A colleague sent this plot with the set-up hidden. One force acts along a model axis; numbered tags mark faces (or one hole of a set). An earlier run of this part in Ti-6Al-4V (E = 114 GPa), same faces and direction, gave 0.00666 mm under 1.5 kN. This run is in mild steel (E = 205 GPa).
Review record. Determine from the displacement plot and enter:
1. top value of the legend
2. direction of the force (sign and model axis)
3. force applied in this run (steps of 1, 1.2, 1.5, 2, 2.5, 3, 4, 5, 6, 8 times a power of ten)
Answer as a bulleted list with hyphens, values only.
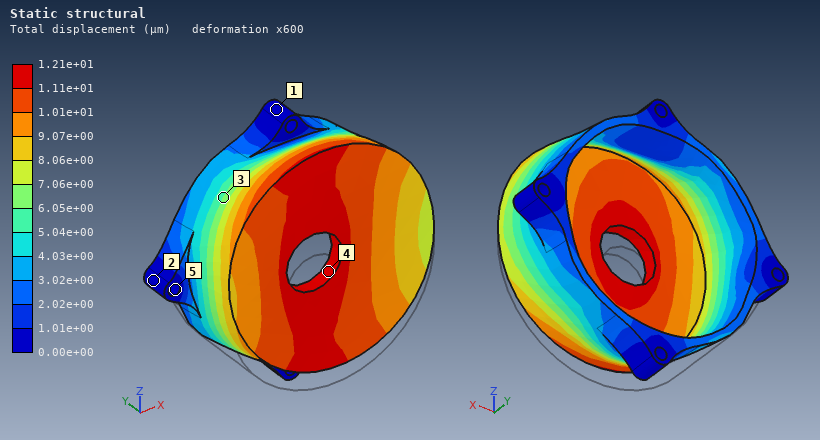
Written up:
- 1.21e+01 µm
- +Z
- 5 kN
